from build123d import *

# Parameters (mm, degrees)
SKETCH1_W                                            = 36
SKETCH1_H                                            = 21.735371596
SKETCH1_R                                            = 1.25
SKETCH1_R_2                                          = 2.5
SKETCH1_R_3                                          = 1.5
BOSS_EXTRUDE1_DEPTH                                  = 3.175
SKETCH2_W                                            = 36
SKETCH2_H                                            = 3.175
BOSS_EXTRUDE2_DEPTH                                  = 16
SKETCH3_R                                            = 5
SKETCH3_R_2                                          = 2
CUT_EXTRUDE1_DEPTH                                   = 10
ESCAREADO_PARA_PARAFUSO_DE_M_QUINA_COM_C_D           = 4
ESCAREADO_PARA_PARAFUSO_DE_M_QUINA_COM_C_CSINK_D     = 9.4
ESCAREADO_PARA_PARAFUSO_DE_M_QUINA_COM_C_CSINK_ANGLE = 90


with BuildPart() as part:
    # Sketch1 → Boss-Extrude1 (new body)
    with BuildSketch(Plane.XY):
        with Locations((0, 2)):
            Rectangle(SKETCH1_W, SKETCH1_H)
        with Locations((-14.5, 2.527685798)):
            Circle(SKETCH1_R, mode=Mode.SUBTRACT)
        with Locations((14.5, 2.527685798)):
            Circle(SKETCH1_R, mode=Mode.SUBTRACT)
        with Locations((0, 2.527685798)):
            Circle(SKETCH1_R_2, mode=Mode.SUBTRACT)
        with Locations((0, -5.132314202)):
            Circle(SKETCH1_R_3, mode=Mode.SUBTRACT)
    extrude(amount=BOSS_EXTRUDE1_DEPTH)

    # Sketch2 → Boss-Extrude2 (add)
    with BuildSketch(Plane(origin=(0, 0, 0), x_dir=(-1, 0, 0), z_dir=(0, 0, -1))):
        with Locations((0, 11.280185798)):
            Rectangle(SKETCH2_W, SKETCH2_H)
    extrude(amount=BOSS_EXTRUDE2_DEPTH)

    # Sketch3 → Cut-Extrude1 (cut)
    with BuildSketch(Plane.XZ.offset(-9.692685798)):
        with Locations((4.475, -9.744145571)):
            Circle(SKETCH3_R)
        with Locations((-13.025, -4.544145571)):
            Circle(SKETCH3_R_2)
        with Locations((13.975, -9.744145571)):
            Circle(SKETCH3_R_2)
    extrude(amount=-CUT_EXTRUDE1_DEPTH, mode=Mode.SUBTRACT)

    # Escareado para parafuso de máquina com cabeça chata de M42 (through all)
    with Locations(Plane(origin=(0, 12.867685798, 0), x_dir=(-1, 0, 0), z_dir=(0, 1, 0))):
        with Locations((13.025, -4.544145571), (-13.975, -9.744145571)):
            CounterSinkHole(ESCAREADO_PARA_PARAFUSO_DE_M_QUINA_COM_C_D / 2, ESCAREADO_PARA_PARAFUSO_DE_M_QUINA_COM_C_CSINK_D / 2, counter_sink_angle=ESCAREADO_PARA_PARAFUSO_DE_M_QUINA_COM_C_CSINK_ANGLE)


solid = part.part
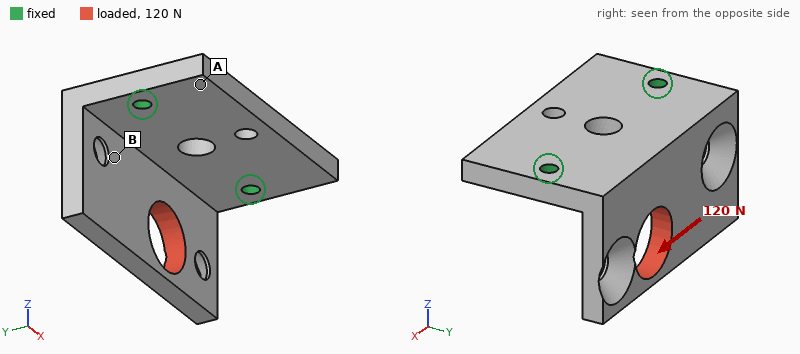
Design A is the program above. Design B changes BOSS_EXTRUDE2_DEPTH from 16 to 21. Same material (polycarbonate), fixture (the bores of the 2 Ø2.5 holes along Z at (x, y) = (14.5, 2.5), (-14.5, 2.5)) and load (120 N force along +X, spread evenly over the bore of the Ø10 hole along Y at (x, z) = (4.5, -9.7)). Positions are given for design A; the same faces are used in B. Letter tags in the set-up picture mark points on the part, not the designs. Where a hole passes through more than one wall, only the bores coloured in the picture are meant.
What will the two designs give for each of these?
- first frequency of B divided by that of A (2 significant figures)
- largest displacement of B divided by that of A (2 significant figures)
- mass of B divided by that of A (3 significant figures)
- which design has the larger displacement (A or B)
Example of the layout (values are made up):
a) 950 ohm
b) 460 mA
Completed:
a) 0.62
b) 1.1
c) 1.15
d) B
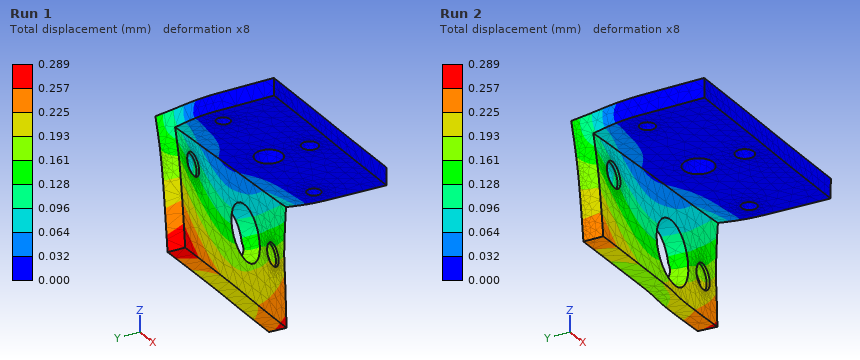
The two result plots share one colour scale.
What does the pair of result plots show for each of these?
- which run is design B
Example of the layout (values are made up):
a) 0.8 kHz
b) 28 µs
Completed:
a) Run 1
